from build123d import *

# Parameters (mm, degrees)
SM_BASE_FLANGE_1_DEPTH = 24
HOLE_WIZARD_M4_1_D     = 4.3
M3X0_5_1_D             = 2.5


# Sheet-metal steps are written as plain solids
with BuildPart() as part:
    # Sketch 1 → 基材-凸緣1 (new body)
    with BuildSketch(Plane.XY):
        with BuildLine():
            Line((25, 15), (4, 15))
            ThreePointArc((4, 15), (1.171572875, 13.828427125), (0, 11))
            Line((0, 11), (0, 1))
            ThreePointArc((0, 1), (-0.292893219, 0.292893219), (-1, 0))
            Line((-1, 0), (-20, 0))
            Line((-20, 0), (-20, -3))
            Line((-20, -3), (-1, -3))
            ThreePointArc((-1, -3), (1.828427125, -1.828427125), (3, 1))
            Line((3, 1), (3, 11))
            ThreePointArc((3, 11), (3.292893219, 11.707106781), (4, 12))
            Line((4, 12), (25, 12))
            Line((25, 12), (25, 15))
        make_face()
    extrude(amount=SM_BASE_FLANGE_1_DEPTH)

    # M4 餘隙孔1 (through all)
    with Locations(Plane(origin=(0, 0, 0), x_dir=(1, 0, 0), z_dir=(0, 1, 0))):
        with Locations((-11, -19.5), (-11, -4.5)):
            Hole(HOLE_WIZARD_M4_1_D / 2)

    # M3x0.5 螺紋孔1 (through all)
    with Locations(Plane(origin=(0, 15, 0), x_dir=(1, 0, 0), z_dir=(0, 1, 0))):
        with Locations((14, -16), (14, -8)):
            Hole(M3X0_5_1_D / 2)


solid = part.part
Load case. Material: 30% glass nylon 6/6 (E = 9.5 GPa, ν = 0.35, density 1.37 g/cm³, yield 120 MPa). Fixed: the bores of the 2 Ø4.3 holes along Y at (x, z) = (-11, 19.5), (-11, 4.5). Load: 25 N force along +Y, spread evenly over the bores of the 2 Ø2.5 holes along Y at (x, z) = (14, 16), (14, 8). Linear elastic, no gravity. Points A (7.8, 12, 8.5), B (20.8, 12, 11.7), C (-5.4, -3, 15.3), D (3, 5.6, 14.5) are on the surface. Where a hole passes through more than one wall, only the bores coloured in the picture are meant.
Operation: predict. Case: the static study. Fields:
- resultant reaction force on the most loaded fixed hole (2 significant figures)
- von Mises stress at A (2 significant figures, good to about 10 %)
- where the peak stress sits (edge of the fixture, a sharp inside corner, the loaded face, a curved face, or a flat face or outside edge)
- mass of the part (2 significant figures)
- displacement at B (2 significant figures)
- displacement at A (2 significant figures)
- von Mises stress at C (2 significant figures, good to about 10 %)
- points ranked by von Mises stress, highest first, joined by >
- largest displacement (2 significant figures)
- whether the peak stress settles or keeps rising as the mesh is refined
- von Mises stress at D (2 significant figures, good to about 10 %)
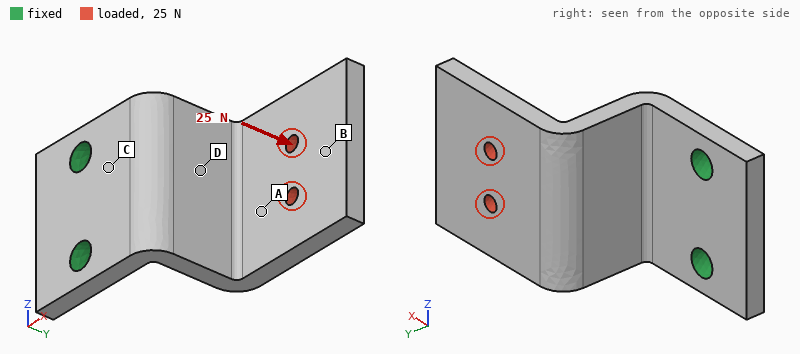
13 N
4.2 MPa
edge of the fixture
5.5 g
0.47 mm
0.24 mm
11 MPa
C > D > A > B
0.57 mm
keeps rising
8.0 MPa
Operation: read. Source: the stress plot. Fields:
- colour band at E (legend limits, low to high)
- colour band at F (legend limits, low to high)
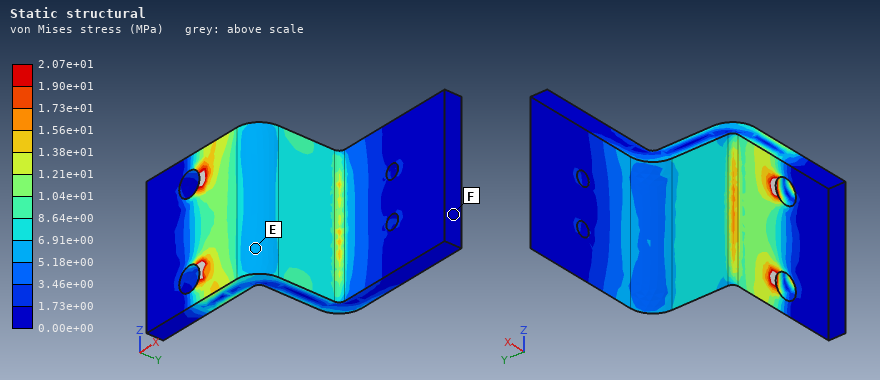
5.18e+00 to 6.91e+00 MPa
0.00e+00 to 1.73e+00 MPa
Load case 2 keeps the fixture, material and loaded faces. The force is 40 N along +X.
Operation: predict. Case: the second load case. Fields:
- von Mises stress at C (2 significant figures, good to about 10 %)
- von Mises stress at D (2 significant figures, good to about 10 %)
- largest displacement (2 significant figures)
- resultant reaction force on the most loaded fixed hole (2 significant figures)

13 MPa
7.6 MPa
0.60 mm
21 N
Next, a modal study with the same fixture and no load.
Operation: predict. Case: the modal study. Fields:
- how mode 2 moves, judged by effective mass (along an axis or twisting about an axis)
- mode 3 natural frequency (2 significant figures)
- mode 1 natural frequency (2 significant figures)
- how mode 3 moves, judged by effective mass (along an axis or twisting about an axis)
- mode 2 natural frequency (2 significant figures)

along Z
2700 Hz
740 Hz
along Z
1900 Hz
